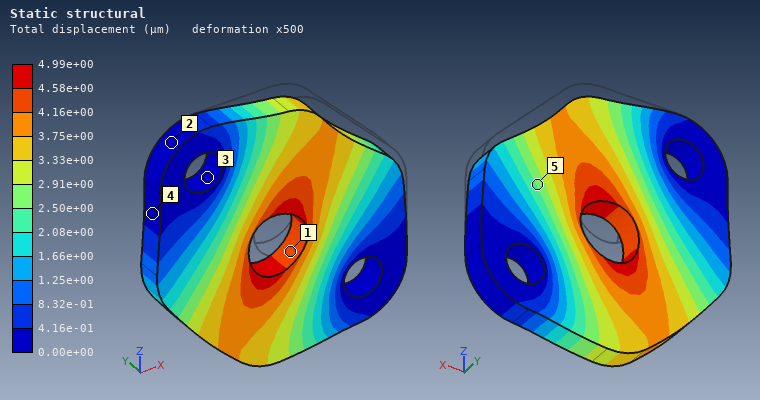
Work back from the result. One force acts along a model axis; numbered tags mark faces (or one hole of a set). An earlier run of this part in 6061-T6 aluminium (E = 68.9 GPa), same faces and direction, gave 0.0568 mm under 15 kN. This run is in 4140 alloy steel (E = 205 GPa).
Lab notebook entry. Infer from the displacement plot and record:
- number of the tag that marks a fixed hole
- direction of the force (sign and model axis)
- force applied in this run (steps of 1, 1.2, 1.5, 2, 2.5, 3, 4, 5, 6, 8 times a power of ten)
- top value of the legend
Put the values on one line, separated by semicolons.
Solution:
3; -Z; 4 kN; 4.99e+00 µm
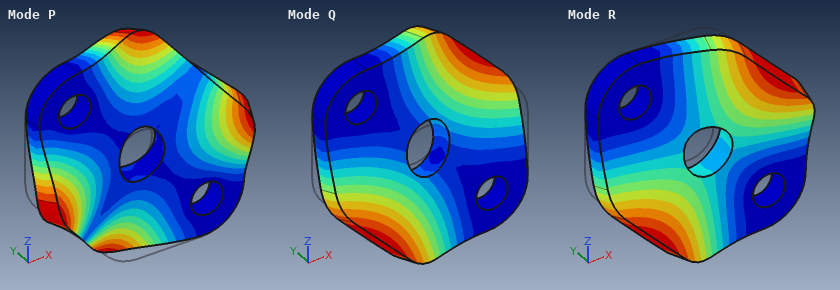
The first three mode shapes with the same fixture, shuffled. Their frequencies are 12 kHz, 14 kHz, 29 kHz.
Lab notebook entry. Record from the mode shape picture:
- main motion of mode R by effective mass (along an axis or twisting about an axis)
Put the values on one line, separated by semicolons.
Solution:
along Y
